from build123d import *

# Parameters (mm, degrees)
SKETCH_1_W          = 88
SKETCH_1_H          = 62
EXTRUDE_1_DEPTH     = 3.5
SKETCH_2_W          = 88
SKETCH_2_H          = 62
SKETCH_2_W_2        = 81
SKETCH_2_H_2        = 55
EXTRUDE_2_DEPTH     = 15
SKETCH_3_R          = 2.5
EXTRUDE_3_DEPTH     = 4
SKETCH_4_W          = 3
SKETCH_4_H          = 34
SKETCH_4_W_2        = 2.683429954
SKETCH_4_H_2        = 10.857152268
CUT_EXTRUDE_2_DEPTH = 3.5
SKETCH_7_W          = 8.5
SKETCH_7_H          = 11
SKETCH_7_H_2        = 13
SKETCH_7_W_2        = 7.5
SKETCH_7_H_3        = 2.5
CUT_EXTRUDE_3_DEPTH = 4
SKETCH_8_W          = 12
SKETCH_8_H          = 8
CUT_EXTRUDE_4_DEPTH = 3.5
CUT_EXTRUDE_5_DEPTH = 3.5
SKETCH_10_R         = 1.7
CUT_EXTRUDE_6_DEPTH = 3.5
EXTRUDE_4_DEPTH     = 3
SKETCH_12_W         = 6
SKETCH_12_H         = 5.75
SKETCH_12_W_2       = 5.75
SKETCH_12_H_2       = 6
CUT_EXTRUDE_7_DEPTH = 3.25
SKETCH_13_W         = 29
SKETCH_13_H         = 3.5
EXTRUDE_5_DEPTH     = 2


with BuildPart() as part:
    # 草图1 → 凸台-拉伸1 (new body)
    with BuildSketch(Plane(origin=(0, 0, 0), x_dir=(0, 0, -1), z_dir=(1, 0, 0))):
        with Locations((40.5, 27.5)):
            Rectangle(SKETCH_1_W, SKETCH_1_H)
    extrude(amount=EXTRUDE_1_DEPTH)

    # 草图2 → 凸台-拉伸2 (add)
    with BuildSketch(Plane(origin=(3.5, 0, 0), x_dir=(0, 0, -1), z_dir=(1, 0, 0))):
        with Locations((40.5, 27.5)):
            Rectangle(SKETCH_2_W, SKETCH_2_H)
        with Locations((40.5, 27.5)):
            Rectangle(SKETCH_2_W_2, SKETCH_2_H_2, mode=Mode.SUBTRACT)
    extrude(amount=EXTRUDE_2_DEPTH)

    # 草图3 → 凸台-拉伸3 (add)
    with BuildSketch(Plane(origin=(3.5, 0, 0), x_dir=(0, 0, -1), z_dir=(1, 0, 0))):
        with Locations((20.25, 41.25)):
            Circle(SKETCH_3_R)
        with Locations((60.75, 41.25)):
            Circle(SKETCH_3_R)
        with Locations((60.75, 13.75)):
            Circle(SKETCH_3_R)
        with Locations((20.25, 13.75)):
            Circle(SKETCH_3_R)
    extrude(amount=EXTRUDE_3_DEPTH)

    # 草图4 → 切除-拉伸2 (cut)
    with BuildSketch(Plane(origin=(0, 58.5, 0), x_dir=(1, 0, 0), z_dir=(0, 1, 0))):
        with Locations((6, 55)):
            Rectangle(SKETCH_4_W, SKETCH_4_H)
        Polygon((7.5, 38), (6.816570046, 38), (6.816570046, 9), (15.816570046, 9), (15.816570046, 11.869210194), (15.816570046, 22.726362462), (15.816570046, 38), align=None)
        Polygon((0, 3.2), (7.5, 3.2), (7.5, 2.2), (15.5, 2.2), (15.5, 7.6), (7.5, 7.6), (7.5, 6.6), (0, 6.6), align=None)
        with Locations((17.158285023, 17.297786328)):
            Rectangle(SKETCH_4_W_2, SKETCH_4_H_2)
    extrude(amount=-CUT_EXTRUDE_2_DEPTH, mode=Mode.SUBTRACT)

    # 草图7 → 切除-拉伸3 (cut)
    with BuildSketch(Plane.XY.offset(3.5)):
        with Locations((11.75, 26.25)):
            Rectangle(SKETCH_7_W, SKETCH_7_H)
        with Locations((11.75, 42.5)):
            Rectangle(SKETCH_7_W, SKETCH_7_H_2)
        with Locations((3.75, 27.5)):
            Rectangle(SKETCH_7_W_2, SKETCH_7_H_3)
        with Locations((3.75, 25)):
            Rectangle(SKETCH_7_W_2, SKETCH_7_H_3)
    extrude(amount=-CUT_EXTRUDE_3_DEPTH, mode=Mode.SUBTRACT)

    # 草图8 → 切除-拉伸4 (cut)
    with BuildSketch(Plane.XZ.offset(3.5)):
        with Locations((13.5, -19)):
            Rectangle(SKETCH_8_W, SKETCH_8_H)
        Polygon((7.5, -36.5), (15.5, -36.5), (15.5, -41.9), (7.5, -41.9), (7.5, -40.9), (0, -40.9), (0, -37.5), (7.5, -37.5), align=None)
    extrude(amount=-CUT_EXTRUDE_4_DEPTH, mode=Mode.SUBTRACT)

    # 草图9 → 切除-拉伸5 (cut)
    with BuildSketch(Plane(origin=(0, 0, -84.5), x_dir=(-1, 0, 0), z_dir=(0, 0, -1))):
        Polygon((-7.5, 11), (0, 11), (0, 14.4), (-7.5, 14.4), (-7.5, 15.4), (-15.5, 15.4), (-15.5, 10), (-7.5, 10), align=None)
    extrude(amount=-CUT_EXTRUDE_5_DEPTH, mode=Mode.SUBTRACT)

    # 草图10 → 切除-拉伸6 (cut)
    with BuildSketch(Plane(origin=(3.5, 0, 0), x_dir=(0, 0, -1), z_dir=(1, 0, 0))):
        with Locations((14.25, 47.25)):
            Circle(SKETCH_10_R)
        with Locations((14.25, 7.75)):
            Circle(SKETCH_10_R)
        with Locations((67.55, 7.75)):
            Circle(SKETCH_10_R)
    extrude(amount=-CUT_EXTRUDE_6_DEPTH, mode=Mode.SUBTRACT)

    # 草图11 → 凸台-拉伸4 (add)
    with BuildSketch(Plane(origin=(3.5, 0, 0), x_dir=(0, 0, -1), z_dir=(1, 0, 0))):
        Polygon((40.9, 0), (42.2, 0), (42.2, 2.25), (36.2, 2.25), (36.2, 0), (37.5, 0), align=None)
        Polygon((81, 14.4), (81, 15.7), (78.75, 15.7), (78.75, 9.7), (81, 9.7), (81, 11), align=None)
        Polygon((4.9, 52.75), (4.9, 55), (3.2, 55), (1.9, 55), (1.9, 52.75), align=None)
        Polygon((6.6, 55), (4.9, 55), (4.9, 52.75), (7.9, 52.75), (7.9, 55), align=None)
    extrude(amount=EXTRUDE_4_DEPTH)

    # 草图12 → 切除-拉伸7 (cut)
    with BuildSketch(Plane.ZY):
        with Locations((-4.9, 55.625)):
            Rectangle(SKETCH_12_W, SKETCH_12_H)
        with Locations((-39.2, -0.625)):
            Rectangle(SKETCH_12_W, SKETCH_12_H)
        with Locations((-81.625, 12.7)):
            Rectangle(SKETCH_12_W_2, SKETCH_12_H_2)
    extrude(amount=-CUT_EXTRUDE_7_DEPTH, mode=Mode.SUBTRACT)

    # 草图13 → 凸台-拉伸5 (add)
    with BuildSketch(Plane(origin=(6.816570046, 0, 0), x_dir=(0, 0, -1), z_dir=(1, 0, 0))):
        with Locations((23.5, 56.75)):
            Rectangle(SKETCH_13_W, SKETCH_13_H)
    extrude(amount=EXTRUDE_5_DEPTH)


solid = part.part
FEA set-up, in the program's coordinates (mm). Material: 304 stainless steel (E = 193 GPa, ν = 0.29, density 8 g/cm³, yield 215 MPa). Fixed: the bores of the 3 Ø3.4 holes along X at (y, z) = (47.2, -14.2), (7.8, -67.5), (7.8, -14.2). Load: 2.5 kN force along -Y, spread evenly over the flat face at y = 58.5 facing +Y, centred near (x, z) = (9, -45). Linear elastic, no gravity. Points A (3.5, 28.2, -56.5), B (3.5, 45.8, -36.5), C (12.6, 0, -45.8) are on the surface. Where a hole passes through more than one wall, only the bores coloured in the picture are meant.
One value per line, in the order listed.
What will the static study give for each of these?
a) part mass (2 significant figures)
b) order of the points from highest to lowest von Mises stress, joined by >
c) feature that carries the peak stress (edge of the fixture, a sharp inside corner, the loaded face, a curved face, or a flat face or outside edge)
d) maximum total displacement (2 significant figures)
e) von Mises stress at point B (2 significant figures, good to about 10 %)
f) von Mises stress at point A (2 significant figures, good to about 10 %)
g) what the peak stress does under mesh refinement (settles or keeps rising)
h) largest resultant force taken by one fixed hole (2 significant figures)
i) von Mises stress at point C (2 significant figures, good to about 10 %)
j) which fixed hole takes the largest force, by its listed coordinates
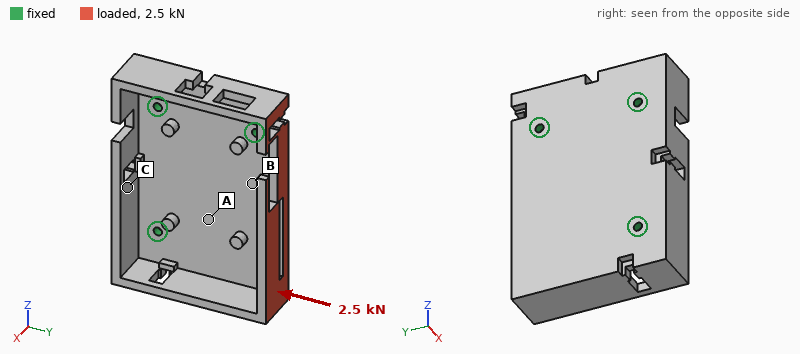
250 g
B > A > C
a sharp inside corner
0.18 mm
53 MPa
30 MPa
keeps rising
1.4 kN
16 MPa
(7.8, -67.5)
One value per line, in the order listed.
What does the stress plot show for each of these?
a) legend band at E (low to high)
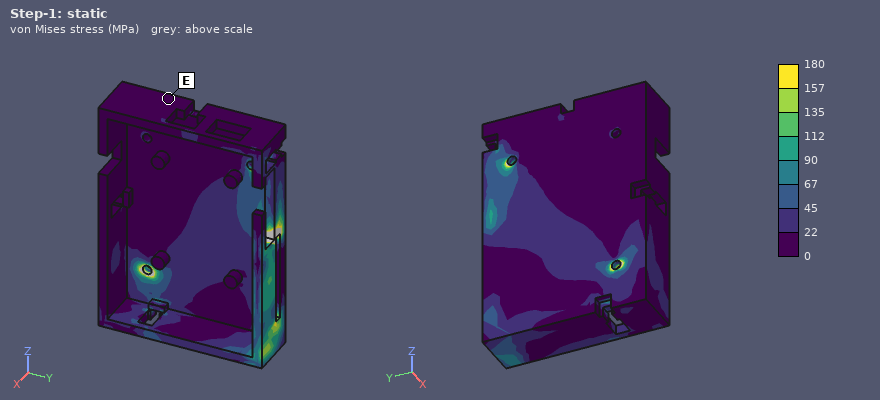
0 to 22 MPa
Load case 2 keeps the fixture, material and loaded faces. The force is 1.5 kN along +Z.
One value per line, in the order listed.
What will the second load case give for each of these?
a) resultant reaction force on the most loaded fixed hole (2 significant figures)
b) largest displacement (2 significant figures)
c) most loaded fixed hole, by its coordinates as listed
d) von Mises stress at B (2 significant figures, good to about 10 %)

1.3 kN
91 µm
(47.2, -14.2)
22 MPa
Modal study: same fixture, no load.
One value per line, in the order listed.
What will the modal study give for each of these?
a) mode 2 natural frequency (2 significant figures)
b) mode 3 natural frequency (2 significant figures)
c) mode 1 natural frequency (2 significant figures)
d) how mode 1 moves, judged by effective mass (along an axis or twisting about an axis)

3900 Hz
4400 Hz
1200 Hz
along X
